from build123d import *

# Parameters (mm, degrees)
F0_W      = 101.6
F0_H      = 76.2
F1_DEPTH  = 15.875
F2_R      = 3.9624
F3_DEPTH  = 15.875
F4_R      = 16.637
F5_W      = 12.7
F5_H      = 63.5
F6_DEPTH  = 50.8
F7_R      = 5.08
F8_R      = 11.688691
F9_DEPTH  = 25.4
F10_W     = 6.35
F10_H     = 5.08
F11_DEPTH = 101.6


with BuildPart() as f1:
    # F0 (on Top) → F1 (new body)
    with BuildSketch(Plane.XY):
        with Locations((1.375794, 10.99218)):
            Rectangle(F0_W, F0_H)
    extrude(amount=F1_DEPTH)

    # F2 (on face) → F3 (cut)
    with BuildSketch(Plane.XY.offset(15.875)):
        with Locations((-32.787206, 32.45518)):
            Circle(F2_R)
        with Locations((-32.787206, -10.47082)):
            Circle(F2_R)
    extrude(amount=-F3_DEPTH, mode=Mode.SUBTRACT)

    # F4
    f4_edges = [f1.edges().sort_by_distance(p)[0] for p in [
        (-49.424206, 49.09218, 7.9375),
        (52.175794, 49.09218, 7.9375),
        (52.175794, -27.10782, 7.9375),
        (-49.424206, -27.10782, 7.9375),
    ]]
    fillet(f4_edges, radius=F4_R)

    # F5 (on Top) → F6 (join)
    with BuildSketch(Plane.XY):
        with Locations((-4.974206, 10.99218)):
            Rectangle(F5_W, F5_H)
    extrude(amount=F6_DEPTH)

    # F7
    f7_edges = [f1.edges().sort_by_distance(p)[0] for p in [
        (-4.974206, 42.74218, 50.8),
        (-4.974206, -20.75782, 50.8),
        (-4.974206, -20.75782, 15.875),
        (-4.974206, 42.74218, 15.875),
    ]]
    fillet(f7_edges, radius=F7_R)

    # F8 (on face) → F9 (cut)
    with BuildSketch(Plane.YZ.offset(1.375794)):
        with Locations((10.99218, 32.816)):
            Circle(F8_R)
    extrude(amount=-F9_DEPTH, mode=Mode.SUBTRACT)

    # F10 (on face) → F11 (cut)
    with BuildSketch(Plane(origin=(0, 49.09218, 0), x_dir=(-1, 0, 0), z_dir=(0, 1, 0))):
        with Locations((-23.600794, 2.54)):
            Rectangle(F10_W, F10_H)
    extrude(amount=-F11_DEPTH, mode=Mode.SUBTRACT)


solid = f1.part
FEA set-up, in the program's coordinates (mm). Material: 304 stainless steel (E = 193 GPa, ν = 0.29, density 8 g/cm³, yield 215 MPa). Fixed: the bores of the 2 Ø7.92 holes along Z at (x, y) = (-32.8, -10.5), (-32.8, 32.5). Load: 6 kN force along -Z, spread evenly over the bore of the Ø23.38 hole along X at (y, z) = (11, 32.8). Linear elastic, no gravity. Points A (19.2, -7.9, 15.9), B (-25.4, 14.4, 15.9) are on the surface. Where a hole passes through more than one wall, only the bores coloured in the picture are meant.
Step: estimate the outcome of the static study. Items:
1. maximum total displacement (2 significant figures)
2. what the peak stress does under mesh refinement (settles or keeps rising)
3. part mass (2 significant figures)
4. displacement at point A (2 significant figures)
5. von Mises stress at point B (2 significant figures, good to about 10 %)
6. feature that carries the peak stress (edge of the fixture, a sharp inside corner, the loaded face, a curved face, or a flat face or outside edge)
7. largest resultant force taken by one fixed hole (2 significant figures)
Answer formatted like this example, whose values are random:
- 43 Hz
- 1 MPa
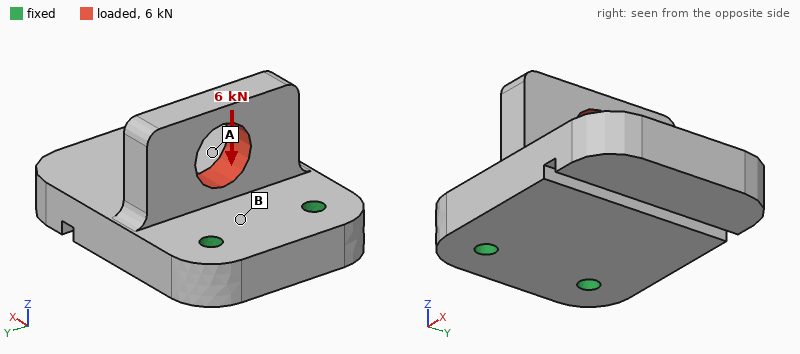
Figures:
- 45 µm
- keeps rising
- 1.1 kg
- 27 µm
- 21 MPa
- edge of the fixture
- 3.0 kN
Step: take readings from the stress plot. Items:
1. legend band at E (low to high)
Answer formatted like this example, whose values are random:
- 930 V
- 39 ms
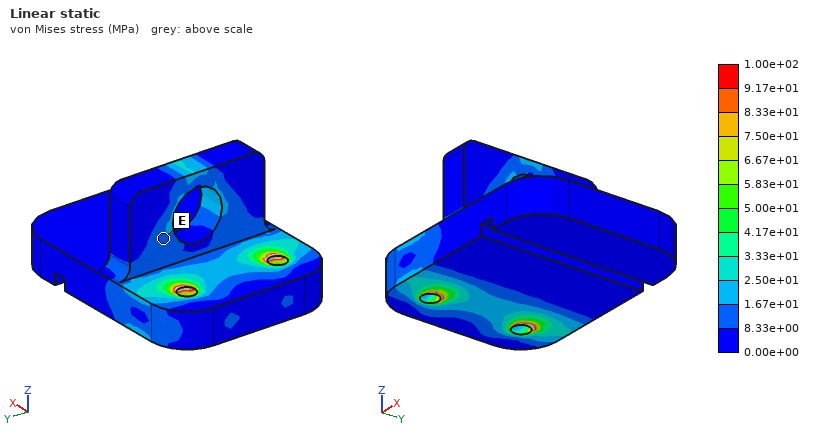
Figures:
- 8.33e+00 to 1.67e+01 MPa
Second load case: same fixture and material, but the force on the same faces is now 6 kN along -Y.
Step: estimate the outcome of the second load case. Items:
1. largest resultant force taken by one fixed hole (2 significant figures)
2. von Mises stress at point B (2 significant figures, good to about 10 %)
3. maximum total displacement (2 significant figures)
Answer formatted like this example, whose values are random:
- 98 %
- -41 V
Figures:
- 5.2 kN
- 22 MPa
- 21 µm
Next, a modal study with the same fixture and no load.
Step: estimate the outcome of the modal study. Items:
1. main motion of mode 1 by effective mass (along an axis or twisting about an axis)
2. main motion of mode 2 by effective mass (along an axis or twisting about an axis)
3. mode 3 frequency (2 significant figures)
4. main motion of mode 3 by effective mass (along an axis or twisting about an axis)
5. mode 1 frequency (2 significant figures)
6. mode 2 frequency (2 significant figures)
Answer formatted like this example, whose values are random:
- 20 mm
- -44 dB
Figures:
- along Z
- twisting about X
- 5100 Hz
- along Y
- 1600 Hz
- 4100 Hz
